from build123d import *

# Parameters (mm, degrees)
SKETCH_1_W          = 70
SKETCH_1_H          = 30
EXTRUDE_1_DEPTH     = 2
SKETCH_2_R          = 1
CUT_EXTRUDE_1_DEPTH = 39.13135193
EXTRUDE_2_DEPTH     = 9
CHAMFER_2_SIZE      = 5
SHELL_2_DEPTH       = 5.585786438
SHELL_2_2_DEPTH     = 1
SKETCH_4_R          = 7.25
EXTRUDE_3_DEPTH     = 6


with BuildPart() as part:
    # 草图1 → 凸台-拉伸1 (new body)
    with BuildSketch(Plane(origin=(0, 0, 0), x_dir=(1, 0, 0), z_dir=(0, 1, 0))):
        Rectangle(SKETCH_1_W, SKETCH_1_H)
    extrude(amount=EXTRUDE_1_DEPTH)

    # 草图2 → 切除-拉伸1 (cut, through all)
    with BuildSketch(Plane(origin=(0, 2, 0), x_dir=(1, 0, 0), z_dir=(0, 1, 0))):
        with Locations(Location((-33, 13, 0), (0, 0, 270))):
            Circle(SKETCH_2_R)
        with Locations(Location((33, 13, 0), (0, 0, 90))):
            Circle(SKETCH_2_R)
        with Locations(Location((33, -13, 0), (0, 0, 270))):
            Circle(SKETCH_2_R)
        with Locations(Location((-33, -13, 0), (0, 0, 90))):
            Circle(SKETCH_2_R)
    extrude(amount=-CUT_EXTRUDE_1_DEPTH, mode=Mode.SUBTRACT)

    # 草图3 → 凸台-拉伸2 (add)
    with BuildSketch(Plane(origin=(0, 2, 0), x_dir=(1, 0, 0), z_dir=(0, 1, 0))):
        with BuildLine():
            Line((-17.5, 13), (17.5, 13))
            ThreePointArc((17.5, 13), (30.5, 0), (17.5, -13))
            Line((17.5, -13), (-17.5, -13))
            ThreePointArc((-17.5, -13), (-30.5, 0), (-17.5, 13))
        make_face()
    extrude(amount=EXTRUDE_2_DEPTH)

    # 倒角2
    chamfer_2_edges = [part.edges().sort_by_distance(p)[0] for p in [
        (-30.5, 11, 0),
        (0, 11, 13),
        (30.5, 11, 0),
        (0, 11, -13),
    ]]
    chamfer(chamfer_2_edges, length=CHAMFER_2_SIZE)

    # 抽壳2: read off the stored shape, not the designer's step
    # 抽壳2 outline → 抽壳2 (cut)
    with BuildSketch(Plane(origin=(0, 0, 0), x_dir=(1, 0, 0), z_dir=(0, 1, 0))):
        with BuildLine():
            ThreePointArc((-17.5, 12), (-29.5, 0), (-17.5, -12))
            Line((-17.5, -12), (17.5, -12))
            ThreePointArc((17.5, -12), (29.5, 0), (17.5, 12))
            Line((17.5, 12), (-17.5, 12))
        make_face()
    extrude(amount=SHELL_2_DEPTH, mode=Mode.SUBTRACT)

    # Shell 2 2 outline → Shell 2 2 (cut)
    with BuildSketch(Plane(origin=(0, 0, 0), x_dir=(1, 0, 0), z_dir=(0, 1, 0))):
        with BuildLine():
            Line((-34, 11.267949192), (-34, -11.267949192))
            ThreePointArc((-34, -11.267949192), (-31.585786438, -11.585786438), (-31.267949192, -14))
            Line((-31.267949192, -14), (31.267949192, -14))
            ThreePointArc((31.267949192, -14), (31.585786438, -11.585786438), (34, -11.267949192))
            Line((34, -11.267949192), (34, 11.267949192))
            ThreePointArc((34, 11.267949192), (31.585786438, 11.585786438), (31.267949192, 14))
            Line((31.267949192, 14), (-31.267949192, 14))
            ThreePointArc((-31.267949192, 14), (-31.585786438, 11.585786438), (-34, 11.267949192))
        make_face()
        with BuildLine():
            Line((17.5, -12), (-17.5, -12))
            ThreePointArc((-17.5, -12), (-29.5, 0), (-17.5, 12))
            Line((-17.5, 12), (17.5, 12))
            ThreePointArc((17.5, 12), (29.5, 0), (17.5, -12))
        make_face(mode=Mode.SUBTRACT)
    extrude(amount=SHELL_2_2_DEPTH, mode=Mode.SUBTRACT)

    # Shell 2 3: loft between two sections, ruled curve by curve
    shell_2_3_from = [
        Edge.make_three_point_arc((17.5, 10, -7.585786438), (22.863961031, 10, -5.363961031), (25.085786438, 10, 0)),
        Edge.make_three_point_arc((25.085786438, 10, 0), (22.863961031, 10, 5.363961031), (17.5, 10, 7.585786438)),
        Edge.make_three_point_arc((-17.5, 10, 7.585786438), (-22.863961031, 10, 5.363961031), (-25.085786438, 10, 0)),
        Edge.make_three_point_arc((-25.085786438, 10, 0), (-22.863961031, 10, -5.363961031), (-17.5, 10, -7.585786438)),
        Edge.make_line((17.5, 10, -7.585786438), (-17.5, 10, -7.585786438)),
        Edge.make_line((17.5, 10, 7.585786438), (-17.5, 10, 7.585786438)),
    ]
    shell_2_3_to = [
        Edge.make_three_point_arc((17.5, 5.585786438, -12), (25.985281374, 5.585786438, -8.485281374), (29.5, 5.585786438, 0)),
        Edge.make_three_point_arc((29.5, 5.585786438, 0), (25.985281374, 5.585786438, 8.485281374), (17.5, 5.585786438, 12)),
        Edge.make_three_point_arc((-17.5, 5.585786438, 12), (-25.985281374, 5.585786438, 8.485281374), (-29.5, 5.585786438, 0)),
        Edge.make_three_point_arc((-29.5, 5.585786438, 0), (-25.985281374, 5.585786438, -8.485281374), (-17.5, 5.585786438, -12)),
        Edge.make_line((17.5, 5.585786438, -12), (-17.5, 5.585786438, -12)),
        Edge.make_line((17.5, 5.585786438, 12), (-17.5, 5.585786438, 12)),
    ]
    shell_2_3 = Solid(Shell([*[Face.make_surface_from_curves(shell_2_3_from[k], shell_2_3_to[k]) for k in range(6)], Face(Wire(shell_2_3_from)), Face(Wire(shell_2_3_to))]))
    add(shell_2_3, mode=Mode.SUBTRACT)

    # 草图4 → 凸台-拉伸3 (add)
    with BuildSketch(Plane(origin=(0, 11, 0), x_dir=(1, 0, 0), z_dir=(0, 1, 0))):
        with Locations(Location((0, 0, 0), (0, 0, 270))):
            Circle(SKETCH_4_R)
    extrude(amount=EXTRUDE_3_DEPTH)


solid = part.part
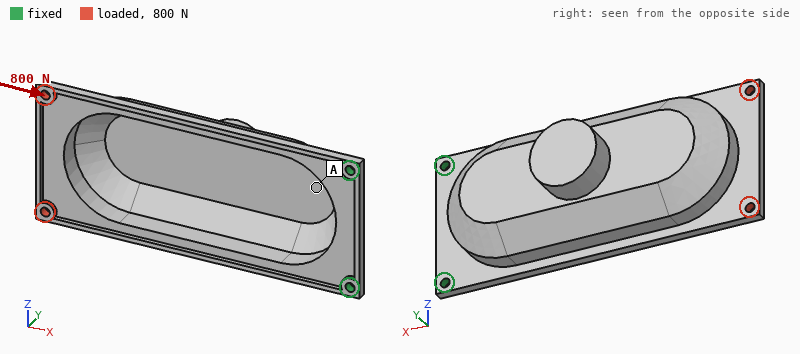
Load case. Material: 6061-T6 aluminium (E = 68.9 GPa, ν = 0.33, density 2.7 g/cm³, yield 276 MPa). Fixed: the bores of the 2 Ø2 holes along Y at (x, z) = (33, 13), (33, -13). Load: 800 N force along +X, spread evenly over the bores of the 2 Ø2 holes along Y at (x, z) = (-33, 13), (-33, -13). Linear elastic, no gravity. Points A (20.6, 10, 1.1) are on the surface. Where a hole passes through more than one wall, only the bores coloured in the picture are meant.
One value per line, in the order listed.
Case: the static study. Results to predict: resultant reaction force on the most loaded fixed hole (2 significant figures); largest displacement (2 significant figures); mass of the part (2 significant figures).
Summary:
400 N
0.61 mm
11 g
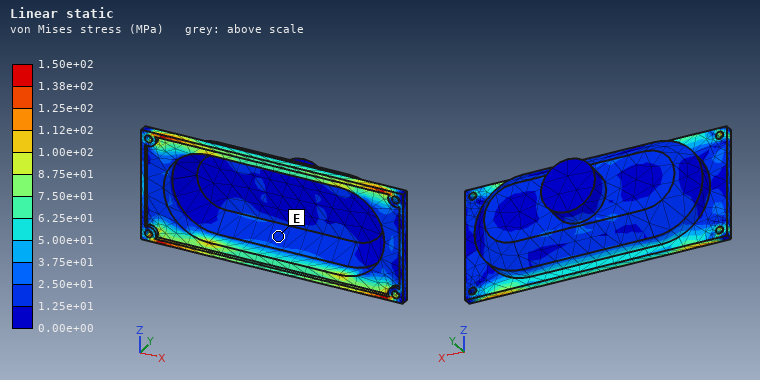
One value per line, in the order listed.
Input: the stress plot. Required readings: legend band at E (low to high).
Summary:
1.25e+01 to 2.50e+01 MPa
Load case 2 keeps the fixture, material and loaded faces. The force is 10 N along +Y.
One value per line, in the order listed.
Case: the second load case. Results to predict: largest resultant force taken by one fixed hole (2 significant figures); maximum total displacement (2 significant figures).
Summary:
17 N
0.80 mm
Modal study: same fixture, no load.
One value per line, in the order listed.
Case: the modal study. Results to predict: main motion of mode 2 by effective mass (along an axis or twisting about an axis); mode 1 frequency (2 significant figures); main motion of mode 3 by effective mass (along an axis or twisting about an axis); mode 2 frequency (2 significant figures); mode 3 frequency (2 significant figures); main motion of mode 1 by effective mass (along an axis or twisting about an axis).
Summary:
along Z
300 Hz
along Z
1000 Hz
2800 Hz
along Y
